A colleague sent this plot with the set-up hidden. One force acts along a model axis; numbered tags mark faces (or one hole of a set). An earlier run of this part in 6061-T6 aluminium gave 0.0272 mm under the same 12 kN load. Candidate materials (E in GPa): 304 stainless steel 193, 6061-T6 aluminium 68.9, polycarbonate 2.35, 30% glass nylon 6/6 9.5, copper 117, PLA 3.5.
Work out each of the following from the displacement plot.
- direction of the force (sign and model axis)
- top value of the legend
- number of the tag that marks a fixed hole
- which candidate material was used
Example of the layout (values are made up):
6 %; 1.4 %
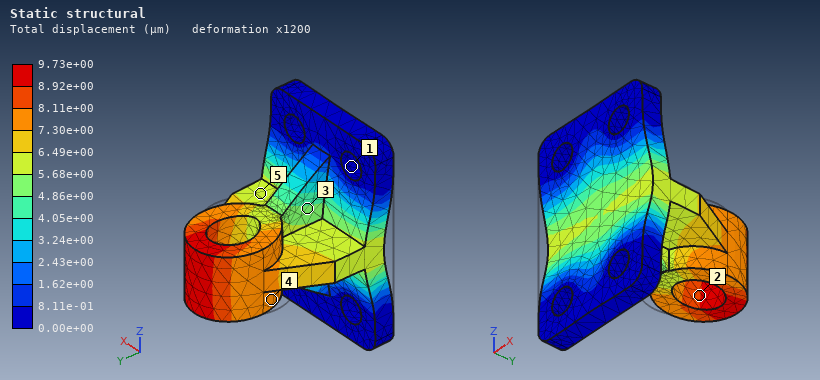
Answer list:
+Y; 9.73e+00 µm; 1; 304 stainless steel
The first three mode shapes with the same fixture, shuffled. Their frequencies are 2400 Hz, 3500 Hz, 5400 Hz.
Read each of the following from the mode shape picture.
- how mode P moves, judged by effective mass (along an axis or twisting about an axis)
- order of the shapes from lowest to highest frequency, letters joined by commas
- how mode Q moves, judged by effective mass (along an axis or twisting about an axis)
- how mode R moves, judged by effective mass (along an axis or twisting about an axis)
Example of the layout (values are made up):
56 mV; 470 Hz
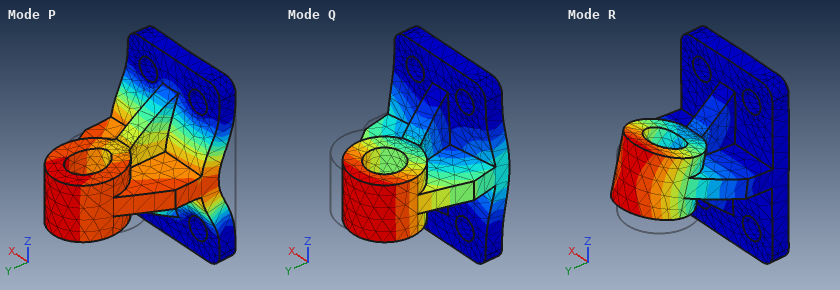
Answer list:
along Y; Q, R, P; along X; along Z
